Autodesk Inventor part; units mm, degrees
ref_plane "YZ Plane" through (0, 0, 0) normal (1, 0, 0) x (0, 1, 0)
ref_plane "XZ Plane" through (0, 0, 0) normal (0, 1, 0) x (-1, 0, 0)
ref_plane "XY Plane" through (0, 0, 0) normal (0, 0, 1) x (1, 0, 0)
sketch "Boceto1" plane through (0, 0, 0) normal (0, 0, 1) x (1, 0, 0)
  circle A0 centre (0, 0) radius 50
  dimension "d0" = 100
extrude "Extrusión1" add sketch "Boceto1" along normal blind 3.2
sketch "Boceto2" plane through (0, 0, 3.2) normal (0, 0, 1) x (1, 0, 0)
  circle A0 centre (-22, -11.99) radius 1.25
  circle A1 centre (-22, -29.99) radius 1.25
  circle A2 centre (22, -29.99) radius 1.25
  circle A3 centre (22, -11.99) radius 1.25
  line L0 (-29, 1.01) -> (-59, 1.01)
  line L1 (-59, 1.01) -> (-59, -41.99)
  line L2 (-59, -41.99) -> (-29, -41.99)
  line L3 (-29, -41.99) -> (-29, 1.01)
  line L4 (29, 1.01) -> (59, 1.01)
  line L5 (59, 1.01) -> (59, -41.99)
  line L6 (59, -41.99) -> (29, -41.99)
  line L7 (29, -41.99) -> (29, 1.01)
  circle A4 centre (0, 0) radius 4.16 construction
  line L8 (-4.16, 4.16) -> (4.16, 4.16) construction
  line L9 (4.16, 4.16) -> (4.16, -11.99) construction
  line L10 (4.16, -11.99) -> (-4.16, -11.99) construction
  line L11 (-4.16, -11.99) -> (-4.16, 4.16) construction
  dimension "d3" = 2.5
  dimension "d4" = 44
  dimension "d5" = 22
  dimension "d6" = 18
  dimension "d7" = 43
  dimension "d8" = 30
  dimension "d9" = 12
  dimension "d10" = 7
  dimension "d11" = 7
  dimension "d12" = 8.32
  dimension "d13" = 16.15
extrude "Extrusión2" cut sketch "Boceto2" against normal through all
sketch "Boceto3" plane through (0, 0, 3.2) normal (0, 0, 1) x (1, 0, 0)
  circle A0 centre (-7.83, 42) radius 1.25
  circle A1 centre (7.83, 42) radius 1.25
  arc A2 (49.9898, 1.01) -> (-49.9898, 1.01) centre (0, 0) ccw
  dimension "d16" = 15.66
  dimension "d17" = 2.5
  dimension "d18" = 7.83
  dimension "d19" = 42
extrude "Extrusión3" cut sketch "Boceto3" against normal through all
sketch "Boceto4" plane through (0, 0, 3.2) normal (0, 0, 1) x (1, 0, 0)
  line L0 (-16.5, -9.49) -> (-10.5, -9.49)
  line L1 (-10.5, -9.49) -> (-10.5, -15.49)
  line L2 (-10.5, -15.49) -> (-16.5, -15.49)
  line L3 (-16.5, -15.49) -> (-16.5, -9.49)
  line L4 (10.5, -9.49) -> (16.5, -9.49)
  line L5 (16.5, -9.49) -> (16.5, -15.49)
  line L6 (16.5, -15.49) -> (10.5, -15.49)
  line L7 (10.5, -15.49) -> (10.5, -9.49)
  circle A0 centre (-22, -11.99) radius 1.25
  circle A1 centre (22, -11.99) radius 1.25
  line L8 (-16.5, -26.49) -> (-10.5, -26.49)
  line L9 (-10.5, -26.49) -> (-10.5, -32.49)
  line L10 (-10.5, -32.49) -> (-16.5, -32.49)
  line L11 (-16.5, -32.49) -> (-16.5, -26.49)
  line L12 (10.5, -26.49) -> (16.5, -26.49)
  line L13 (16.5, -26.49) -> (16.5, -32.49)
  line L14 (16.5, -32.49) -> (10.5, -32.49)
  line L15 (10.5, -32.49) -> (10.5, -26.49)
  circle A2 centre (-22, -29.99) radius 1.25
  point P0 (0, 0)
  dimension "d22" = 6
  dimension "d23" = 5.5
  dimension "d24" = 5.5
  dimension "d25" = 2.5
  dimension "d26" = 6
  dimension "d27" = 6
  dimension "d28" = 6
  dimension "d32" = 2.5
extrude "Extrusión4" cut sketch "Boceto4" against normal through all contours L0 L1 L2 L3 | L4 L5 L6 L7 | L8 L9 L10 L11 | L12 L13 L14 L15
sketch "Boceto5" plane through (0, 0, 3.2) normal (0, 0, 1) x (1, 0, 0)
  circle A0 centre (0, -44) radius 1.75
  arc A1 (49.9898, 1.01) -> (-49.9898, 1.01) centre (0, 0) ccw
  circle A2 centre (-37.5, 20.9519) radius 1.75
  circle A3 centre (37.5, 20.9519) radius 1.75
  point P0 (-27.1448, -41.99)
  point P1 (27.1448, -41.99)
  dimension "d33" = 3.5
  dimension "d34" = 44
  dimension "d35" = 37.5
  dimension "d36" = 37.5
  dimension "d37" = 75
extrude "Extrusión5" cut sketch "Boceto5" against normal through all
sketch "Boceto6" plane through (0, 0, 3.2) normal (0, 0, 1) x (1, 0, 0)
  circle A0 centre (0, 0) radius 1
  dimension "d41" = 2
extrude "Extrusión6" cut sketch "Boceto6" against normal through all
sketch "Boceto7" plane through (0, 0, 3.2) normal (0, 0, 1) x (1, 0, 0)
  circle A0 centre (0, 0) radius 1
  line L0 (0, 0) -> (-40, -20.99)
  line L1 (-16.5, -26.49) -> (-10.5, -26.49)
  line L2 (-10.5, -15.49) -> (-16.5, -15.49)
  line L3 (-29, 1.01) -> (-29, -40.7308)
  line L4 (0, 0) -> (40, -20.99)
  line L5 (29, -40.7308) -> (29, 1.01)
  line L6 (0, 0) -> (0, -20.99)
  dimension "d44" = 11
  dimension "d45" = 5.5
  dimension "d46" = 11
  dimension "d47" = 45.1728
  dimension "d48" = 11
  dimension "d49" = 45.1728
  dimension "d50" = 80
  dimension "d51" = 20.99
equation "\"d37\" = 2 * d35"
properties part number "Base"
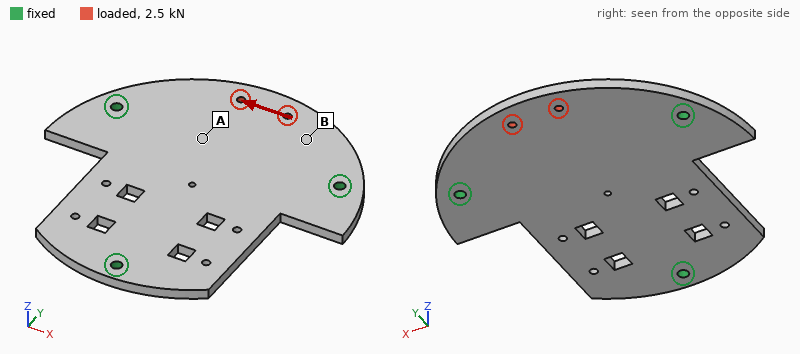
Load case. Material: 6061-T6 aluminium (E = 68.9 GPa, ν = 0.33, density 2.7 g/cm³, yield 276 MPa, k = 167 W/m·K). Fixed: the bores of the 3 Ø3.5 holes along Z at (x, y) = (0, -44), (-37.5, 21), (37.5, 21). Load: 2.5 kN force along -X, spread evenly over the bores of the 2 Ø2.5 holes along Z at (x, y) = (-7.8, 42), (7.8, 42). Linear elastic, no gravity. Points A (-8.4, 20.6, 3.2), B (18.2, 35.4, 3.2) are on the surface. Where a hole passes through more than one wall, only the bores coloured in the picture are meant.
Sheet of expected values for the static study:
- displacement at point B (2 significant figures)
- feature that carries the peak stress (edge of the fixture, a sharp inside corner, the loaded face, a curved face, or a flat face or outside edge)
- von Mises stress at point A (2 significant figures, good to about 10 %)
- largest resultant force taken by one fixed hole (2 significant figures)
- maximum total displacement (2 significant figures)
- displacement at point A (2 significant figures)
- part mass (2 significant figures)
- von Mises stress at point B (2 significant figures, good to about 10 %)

10 µm
the loaded face
7.3 MPa
1.4 kN
18 µm
5.9 µm
55 g
22 MPa
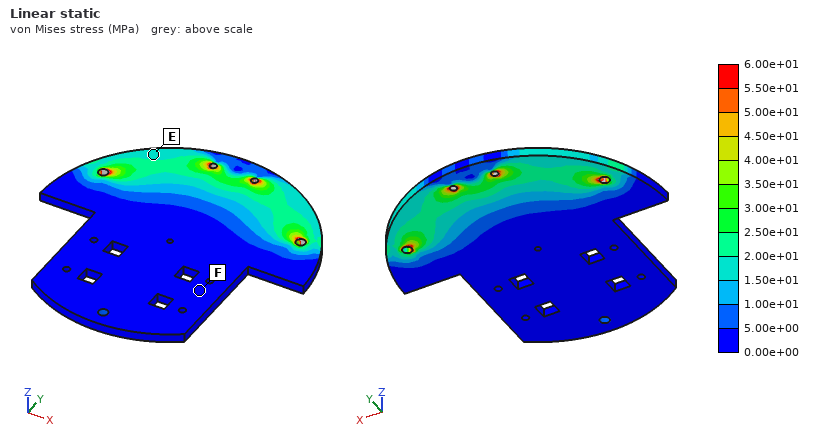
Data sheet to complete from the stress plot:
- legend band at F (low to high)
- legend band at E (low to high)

0.00e+00 to 5.00e+00 MPa
1.50e+01 to 2.00e+01 MPa
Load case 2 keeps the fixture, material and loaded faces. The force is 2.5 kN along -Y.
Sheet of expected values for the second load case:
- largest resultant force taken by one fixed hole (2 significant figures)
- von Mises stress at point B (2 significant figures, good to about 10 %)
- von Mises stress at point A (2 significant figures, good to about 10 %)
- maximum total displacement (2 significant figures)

880 N
16 MPa
14 MPa
18 µm
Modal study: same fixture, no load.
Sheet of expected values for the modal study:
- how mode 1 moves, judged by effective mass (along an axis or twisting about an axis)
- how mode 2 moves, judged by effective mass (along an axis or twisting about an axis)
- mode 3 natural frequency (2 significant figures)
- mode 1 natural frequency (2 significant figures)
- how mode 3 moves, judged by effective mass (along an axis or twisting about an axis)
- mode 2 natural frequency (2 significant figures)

along Z
along Z
2900 Hz
2000 Hz
twisting about Y
2500 Hz
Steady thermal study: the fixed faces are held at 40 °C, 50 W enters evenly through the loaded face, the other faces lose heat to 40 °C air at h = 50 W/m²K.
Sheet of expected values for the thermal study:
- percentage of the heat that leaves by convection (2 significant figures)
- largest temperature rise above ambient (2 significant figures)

23 %
66 K
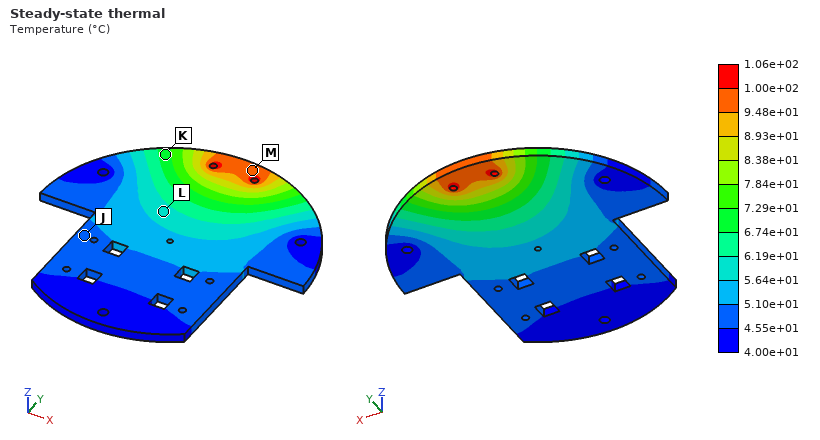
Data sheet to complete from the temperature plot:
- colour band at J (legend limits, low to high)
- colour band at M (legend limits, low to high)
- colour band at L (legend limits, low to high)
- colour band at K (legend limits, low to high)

4.55e+01 to 5.10e+01 °C
9.48e+01 to 1.00e+02 °C
5.64e+01 to 6.19e+01 °C
6.74e+01 to 7.29e+01 °C
